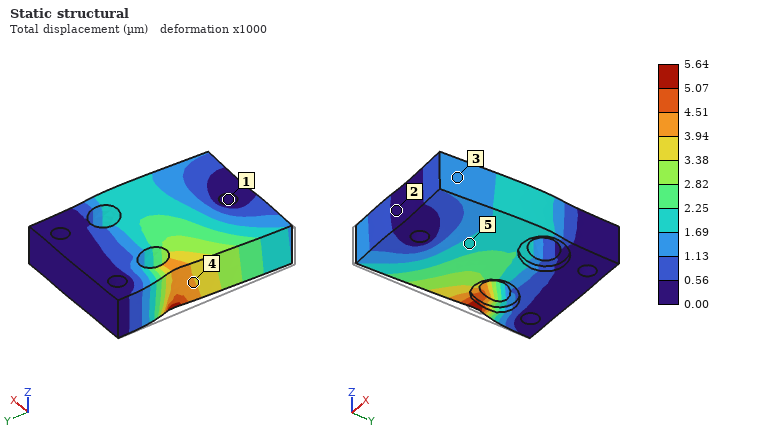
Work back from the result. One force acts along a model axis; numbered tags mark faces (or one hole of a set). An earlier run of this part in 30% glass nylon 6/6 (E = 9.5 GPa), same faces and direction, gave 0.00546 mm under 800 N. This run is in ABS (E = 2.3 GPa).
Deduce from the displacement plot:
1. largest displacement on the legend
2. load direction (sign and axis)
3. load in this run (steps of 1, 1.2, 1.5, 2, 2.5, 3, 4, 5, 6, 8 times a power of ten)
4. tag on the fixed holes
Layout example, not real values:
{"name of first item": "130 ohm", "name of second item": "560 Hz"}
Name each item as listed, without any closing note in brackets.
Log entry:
{"largest displacement on the legend": "5.64 µm", "load direction": "+X", "load in this run": "200 N", "tag on the fixed holes": "1"}
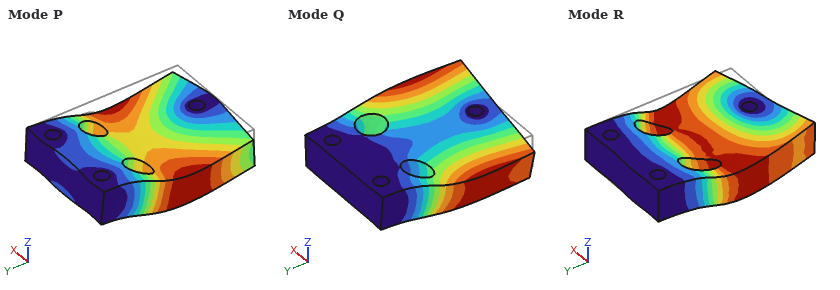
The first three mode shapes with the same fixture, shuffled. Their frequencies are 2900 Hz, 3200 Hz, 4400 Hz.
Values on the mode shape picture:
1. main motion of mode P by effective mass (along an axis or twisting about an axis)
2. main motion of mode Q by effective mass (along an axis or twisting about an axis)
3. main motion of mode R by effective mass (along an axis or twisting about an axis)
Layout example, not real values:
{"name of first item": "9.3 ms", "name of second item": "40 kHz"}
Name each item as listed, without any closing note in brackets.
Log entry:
{"main motion of mode P by effective mass": "along Z", "main motion of mode Q by effective mass": "twisting about Y", "main motion of mode R by effective mass": "along X"}
